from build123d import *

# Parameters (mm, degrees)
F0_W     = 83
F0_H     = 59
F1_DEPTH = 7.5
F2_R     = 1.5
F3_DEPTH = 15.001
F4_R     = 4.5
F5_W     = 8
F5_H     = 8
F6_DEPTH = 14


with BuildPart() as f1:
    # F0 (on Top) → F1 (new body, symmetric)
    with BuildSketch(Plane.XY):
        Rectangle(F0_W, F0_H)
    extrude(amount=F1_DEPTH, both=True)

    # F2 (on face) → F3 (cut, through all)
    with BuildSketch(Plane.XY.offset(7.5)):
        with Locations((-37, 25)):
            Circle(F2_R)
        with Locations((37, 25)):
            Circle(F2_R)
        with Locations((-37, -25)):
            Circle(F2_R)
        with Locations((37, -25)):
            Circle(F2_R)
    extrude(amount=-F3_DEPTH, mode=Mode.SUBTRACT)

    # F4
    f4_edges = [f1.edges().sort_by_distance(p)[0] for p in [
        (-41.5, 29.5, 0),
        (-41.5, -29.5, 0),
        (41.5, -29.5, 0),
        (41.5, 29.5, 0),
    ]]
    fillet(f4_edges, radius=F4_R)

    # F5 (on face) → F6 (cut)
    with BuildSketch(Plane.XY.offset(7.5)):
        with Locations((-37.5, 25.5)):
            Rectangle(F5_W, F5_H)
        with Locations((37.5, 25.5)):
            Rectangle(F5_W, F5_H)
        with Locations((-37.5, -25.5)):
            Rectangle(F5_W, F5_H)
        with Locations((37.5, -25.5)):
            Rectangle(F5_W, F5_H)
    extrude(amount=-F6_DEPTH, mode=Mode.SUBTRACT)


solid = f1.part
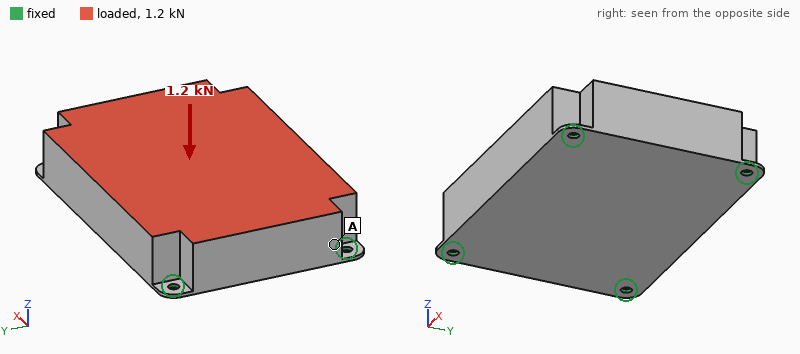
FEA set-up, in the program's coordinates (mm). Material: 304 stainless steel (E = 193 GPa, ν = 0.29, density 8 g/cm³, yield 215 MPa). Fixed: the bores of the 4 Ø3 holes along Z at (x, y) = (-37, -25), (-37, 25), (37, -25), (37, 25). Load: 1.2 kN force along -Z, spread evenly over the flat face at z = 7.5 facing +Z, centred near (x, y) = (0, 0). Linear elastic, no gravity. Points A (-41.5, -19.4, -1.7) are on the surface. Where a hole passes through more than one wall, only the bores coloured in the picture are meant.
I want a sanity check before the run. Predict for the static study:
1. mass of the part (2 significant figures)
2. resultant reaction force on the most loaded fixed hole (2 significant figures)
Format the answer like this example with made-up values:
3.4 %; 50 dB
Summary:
560 g; 360 N
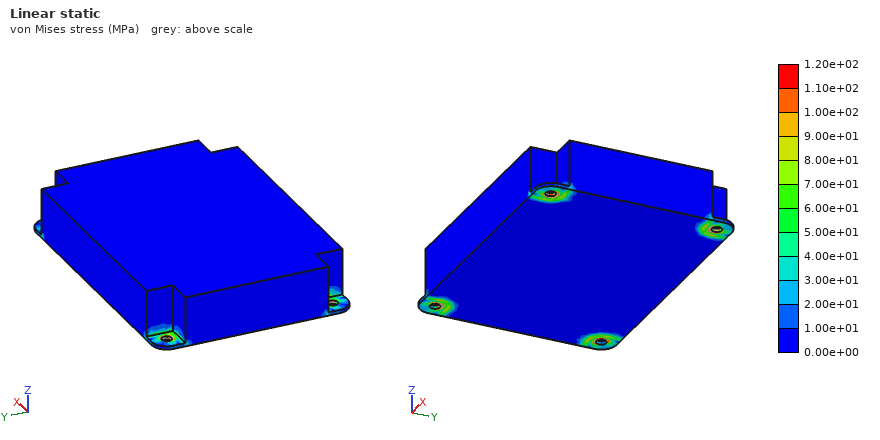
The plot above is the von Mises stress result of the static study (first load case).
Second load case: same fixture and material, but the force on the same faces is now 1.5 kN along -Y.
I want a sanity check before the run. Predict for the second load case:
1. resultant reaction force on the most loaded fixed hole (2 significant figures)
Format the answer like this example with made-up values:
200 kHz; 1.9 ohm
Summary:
460 N
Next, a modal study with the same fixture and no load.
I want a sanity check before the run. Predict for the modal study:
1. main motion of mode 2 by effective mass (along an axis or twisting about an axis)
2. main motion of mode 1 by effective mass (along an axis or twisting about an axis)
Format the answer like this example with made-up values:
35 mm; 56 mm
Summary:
along Y; along Z
